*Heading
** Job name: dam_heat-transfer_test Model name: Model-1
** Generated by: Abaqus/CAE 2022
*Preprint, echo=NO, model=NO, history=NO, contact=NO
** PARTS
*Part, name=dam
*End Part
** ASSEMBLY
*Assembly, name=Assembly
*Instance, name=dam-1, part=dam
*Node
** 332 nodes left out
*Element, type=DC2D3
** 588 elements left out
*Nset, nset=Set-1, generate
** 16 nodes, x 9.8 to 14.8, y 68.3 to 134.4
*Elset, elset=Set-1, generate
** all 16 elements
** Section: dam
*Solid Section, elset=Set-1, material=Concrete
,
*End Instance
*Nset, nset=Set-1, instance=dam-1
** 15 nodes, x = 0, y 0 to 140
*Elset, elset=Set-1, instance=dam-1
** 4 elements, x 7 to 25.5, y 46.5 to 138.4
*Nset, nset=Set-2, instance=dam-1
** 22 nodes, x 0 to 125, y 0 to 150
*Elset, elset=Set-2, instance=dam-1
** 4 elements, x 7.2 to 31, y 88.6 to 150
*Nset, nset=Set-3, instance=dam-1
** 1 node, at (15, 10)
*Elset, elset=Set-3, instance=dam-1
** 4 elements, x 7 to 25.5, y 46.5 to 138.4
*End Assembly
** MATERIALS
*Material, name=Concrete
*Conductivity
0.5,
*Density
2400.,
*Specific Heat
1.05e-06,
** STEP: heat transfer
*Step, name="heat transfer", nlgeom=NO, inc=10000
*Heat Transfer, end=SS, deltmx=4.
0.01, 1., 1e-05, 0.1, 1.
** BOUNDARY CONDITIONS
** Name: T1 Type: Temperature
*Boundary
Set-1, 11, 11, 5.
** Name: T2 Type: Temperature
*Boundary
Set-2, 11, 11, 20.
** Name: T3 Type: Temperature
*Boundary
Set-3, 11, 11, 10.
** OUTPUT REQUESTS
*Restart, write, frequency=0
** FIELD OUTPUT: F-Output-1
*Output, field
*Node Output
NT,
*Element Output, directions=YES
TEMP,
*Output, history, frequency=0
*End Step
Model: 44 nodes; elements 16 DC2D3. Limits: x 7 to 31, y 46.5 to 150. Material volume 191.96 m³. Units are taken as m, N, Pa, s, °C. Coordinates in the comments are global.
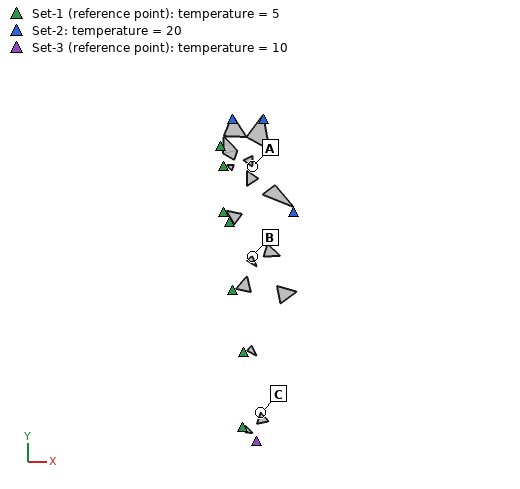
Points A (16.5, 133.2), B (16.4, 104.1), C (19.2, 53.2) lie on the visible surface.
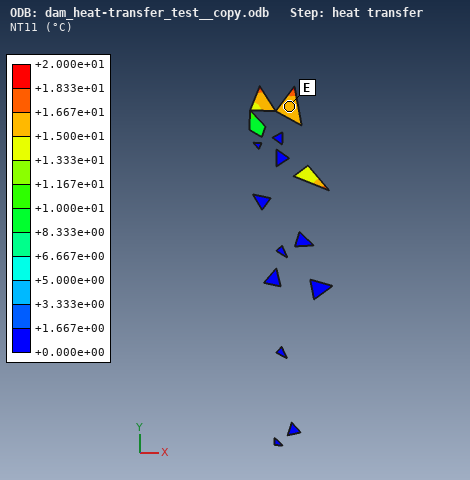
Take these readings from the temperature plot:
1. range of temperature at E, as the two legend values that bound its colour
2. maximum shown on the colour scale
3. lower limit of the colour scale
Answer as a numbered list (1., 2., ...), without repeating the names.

1. +1.500e+01 to +1.667e+01 °C
2. +2.000e+01 °C
3. +0.000e+00 °C
